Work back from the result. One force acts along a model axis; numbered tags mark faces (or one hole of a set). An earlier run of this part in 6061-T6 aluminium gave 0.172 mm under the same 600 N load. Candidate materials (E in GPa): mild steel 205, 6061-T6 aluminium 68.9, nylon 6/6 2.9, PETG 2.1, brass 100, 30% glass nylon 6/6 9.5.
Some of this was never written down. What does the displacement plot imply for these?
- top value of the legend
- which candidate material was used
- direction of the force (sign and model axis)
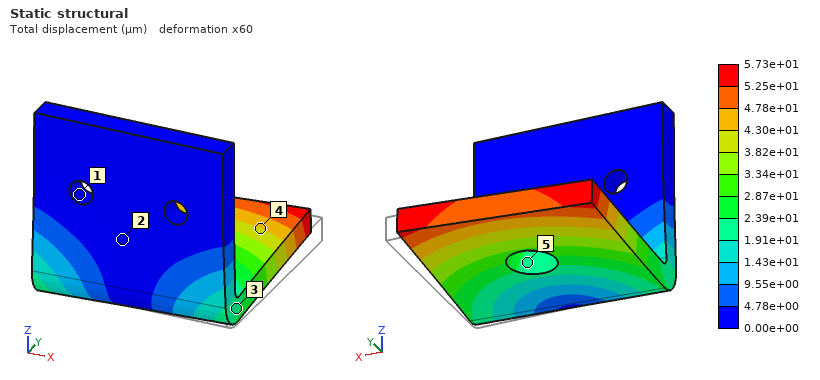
5.73e+01 µm
mild steel
-X
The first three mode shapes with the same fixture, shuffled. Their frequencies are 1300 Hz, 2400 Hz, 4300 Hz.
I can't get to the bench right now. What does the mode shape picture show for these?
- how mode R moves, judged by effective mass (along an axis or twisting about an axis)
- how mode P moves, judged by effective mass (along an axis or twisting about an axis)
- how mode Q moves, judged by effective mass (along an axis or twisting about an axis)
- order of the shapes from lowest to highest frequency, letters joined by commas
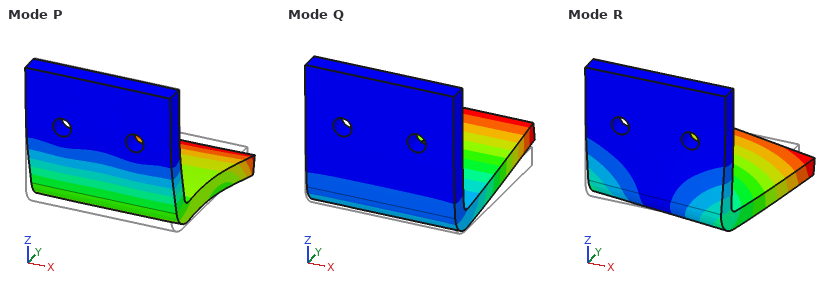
along X
along Y
along Z
Q, R, P
